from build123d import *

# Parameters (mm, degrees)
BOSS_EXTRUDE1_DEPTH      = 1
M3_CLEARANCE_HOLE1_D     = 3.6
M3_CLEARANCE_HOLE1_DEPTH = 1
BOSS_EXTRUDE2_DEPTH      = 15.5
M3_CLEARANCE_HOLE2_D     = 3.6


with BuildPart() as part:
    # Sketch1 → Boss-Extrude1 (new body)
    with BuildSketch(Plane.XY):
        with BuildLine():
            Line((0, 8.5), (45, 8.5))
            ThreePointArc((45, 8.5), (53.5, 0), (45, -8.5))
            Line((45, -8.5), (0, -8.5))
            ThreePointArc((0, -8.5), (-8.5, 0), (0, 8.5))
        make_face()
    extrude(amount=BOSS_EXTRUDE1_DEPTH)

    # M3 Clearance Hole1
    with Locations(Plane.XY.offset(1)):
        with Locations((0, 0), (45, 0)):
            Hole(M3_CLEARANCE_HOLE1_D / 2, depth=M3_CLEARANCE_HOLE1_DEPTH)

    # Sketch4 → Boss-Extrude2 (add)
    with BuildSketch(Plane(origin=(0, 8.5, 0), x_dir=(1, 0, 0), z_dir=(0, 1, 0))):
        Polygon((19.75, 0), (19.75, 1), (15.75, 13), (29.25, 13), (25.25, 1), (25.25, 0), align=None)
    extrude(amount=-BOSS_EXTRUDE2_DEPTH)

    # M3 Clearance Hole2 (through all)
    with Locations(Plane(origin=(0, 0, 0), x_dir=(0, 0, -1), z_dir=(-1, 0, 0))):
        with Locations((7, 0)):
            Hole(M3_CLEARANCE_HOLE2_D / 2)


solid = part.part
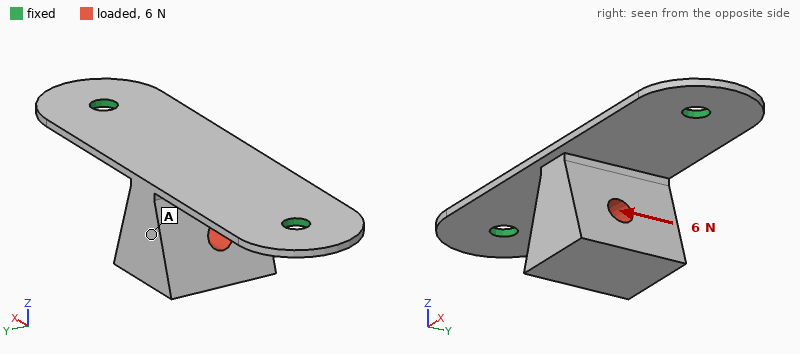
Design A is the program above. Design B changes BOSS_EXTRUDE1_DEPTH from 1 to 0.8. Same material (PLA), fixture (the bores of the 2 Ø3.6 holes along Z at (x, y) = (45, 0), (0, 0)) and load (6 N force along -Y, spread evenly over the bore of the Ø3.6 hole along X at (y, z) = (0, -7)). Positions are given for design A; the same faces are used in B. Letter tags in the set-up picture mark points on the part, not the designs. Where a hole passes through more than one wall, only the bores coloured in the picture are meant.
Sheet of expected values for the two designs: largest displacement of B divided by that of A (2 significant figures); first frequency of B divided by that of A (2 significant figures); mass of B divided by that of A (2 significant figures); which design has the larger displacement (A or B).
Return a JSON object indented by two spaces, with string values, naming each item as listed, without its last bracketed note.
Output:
{
  "largest displacement of B divided by that of A": "1.9",
  "first frequency of B divided by that of A": "0.74",
  "mass of B divided by that of A": "0.93",
  "which design has the larger displacement": "B"
}
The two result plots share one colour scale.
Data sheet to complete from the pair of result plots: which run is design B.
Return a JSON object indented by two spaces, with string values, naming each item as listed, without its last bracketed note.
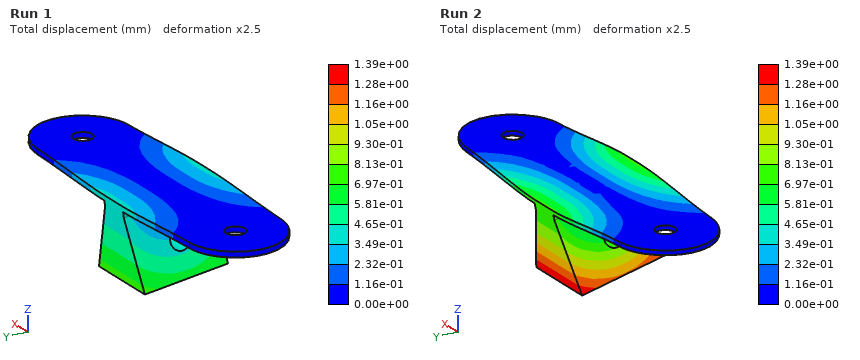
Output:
{
  "which run is design B": "Run 2"
}
